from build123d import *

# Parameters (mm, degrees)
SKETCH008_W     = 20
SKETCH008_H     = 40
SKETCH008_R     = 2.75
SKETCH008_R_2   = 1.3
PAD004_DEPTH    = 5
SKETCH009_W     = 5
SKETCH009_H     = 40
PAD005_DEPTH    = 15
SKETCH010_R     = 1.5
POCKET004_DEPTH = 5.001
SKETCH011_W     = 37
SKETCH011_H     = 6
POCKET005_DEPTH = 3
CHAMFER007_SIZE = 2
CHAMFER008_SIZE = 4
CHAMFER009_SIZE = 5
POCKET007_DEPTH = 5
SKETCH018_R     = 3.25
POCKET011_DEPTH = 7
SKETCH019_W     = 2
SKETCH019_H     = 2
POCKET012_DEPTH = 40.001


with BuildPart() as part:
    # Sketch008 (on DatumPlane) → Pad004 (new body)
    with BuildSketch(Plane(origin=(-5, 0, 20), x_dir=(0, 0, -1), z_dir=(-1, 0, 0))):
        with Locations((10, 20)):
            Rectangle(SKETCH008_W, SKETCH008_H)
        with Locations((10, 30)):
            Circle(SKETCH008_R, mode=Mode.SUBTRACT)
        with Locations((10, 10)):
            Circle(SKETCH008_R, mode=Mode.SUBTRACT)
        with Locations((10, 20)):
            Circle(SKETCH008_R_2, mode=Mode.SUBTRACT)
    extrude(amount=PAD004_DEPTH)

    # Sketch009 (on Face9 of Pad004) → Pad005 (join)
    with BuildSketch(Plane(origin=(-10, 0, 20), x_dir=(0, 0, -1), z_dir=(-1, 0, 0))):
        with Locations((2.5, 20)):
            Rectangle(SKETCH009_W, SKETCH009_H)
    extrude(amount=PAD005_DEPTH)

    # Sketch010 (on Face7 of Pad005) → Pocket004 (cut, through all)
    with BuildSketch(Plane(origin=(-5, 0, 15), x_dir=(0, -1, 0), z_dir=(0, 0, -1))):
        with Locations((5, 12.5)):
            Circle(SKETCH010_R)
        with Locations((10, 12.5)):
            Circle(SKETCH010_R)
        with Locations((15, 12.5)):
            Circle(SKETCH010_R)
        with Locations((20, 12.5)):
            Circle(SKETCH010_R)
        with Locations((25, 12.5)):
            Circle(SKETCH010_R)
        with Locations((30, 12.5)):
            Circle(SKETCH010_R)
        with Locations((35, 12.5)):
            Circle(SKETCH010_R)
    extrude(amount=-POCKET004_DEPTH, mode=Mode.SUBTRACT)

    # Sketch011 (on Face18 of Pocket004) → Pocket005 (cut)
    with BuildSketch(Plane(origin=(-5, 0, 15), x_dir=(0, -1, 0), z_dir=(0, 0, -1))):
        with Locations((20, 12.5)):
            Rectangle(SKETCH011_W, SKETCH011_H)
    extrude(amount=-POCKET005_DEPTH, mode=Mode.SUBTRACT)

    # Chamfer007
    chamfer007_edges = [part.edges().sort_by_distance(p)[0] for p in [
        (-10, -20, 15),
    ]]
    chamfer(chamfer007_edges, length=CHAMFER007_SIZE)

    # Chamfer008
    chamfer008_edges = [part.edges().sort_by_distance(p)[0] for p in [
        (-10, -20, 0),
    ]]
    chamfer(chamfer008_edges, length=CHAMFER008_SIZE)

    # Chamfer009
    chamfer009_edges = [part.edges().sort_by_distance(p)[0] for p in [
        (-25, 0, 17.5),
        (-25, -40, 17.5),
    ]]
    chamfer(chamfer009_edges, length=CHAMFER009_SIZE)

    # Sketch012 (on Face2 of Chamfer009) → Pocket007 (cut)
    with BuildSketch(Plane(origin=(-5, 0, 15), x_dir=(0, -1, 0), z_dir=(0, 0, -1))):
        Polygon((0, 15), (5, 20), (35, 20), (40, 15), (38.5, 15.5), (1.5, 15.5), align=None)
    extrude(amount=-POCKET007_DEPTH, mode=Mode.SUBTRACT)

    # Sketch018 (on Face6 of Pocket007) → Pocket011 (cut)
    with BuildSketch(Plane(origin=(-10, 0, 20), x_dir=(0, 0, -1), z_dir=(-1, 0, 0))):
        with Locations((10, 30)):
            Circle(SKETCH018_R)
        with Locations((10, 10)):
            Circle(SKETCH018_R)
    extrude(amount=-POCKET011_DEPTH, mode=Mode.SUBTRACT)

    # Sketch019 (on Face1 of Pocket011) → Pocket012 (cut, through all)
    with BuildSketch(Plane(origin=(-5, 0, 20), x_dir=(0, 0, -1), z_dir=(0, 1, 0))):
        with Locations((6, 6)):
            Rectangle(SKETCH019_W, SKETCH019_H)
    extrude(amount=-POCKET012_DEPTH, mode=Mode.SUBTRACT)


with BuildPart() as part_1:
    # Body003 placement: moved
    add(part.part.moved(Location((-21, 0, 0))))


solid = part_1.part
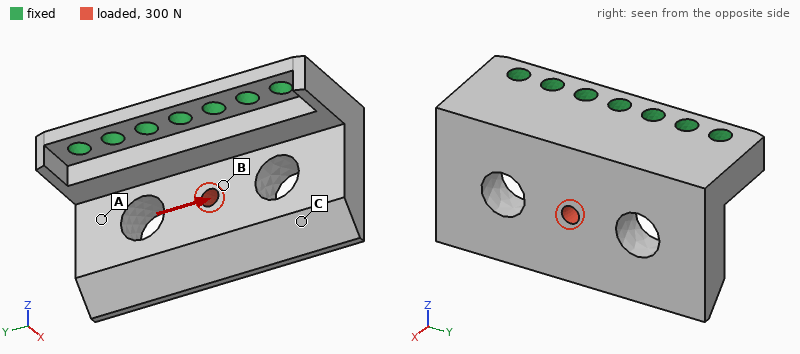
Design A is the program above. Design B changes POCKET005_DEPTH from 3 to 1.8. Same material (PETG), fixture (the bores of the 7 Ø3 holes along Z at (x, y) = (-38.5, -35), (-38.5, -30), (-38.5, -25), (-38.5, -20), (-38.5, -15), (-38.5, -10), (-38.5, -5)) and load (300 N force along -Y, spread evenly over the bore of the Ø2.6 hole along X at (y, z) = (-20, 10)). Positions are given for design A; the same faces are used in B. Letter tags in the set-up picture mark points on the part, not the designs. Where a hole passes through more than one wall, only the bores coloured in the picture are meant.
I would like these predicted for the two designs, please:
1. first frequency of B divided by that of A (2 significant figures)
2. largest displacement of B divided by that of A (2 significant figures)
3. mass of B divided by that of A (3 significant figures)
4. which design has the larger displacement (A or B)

1.7
0.70
1.04
A
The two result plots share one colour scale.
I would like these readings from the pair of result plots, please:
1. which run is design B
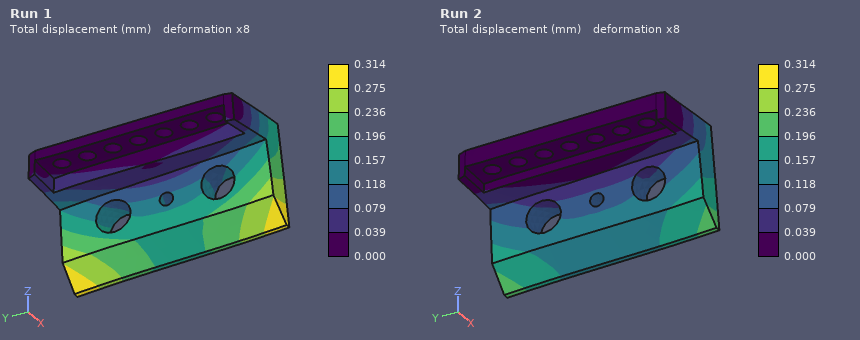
Run 2
